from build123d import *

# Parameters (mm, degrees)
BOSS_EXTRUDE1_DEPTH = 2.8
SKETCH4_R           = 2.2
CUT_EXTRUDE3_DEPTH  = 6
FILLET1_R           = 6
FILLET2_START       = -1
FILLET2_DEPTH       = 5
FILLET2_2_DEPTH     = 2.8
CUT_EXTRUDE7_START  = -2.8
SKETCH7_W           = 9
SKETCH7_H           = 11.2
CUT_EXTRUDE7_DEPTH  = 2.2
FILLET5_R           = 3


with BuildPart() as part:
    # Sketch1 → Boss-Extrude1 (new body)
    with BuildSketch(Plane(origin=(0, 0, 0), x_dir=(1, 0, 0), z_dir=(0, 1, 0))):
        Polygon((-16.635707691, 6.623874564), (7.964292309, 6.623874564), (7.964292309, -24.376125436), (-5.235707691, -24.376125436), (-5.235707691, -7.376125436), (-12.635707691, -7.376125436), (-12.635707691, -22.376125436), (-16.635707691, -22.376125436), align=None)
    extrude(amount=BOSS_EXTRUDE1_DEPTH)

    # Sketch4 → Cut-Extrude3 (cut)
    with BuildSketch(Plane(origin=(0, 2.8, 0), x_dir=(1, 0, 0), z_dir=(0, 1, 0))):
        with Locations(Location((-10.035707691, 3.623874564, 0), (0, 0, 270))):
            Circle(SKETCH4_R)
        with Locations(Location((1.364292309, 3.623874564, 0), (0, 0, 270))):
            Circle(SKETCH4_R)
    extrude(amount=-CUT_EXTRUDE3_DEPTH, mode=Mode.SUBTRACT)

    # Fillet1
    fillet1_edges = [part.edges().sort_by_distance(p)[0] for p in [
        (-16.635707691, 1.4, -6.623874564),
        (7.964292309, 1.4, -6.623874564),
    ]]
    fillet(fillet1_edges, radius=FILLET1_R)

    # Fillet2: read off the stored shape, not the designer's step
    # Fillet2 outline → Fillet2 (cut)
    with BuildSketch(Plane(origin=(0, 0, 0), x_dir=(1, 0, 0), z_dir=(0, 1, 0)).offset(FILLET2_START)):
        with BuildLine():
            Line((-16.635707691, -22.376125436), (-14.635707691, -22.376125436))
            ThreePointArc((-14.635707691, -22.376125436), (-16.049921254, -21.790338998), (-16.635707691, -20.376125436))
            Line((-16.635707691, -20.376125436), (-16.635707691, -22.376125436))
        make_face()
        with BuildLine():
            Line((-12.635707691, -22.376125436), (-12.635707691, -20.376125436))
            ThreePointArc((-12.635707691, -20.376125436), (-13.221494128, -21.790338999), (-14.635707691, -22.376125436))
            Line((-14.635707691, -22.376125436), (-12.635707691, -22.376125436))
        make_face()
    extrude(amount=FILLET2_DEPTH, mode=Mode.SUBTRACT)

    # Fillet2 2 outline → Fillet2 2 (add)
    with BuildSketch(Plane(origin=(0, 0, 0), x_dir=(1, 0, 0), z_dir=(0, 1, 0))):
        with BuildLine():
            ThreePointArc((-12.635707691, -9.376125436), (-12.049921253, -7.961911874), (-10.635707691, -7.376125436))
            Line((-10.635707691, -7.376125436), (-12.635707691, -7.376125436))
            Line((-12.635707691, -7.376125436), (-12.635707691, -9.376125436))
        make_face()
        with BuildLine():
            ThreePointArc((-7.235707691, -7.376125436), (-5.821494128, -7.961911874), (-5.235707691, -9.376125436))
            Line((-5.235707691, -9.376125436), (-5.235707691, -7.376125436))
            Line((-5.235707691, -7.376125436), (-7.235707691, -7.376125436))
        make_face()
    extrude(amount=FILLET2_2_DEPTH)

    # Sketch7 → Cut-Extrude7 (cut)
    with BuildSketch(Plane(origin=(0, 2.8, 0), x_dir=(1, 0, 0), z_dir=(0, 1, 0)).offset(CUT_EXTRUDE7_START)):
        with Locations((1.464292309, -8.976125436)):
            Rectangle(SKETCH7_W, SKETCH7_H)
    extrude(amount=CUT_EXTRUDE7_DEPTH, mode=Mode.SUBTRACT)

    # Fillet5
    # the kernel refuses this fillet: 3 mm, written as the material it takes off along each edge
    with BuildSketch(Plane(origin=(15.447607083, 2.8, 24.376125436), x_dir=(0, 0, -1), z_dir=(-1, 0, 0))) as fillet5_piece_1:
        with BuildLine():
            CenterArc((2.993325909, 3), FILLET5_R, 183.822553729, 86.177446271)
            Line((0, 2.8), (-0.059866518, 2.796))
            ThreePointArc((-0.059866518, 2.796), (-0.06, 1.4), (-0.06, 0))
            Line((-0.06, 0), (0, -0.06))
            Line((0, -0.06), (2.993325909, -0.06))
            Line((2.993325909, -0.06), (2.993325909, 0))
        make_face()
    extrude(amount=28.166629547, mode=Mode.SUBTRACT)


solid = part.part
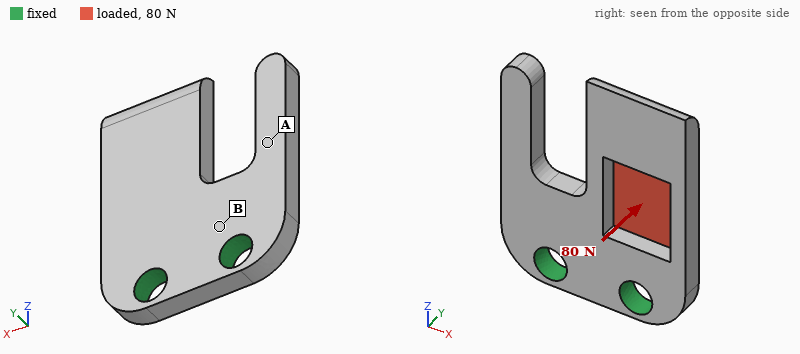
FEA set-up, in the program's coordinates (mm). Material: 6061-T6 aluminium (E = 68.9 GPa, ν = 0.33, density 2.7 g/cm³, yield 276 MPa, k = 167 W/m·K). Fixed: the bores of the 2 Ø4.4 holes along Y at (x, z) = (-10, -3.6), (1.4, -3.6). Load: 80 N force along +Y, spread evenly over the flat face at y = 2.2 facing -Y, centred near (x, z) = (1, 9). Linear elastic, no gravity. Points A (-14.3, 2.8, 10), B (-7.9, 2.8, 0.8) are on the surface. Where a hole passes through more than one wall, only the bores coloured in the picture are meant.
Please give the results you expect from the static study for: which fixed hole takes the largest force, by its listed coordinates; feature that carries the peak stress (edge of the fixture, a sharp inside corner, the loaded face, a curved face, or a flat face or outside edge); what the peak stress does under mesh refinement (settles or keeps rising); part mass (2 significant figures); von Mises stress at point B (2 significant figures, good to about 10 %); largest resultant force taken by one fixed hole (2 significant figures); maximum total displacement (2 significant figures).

(1.4, -3.6)
edge of the fixture
keeps rising
3.7 g
18 MPa
71 N
85 µm
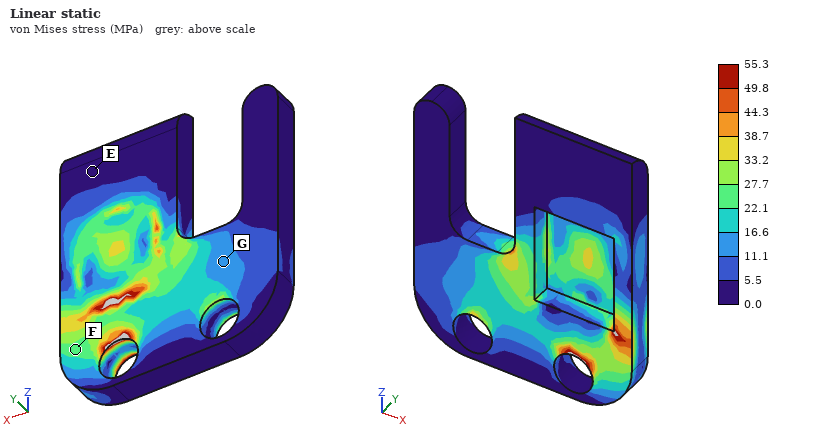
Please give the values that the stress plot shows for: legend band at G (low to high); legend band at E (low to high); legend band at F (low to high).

11.1 to 16.6 MPa
0.0 to 5.5 MPa
22.1 to 27.7 MPa
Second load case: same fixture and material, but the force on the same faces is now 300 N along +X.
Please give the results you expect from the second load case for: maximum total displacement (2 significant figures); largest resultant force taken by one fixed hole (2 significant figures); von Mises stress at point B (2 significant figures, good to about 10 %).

18 µm
280 N
18 MPa
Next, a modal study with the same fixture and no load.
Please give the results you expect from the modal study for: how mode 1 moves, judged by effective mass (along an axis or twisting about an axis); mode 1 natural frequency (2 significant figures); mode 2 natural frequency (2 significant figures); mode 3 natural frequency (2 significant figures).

along Y
3200 Hz
5500 Hz
9500 Hz
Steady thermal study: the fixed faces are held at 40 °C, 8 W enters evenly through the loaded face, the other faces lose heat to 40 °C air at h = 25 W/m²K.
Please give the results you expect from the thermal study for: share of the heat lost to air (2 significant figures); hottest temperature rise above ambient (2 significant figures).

4.0 %
22 K
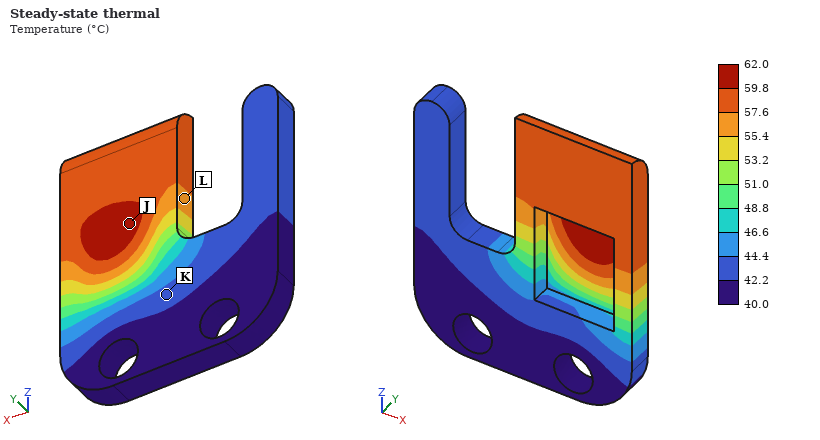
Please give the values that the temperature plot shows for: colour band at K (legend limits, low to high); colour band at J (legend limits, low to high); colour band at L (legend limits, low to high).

42.2 to 44.4 °C
59.8 to 62.0 °C
55.4 to 57.6 °C
